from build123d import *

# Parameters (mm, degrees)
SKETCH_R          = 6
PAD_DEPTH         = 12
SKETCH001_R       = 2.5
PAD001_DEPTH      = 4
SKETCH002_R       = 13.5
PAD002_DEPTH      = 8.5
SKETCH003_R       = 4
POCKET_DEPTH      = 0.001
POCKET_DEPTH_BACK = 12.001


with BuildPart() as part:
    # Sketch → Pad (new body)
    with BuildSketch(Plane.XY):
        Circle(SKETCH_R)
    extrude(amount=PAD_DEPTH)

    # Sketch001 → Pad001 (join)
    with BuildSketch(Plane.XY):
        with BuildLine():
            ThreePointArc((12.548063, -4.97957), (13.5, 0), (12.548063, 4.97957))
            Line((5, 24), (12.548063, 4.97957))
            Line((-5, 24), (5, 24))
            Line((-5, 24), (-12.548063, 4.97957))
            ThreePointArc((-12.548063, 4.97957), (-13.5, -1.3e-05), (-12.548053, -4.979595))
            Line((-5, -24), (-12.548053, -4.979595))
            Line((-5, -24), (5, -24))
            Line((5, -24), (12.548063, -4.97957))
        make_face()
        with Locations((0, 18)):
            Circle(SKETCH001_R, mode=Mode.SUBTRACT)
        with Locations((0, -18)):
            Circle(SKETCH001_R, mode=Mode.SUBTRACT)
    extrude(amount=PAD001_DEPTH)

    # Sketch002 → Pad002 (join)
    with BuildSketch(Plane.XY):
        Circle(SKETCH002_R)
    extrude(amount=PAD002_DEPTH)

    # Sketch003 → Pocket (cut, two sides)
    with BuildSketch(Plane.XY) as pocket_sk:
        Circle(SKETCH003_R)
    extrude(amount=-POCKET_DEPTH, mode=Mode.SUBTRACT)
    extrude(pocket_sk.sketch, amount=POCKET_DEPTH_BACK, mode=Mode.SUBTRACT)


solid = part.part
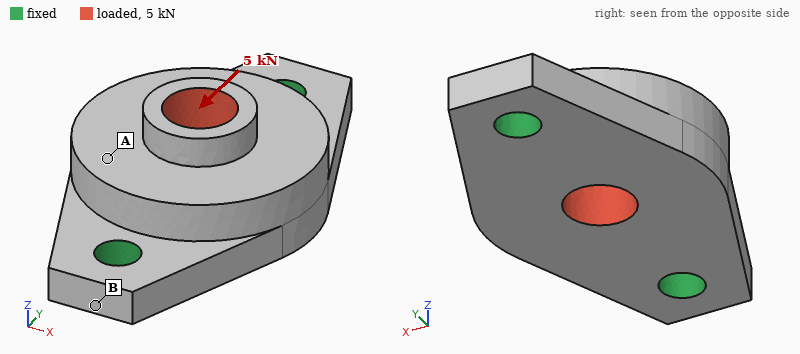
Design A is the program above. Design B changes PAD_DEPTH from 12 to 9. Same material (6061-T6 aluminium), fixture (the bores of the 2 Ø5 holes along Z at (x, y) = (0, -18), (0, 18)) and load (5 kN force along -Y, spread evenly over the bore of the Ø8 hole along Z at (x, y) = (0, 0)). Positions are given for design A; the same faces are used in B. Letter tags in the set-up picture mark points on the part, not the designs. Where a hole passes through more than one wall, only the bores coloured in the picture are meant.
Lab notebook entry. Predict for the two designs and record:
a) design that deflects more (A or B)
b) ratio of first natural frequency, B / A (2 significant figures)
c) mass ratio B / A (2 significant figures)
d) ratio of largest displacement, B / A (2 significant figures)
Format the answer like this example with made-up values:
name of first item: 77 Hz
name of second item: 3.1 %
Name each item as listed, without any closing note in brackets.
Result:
design that deflects more: A
ratio of first natural frequency, B / A: 1.0
mass ratio B / A: 0.97
ratio of largest displacement, B / A: 0.57
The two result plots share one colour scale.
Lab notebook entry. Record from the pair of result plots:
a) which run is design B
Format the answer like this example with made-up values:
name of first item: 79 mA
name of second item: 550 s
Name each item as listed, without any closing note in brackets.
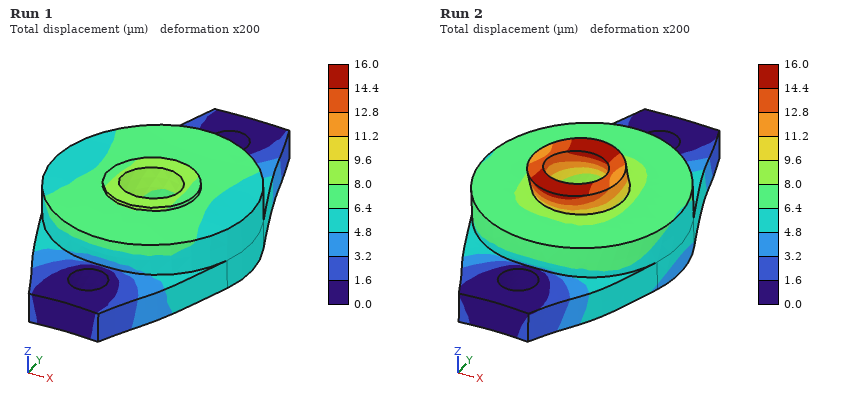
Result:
which run is design B: Run 1
